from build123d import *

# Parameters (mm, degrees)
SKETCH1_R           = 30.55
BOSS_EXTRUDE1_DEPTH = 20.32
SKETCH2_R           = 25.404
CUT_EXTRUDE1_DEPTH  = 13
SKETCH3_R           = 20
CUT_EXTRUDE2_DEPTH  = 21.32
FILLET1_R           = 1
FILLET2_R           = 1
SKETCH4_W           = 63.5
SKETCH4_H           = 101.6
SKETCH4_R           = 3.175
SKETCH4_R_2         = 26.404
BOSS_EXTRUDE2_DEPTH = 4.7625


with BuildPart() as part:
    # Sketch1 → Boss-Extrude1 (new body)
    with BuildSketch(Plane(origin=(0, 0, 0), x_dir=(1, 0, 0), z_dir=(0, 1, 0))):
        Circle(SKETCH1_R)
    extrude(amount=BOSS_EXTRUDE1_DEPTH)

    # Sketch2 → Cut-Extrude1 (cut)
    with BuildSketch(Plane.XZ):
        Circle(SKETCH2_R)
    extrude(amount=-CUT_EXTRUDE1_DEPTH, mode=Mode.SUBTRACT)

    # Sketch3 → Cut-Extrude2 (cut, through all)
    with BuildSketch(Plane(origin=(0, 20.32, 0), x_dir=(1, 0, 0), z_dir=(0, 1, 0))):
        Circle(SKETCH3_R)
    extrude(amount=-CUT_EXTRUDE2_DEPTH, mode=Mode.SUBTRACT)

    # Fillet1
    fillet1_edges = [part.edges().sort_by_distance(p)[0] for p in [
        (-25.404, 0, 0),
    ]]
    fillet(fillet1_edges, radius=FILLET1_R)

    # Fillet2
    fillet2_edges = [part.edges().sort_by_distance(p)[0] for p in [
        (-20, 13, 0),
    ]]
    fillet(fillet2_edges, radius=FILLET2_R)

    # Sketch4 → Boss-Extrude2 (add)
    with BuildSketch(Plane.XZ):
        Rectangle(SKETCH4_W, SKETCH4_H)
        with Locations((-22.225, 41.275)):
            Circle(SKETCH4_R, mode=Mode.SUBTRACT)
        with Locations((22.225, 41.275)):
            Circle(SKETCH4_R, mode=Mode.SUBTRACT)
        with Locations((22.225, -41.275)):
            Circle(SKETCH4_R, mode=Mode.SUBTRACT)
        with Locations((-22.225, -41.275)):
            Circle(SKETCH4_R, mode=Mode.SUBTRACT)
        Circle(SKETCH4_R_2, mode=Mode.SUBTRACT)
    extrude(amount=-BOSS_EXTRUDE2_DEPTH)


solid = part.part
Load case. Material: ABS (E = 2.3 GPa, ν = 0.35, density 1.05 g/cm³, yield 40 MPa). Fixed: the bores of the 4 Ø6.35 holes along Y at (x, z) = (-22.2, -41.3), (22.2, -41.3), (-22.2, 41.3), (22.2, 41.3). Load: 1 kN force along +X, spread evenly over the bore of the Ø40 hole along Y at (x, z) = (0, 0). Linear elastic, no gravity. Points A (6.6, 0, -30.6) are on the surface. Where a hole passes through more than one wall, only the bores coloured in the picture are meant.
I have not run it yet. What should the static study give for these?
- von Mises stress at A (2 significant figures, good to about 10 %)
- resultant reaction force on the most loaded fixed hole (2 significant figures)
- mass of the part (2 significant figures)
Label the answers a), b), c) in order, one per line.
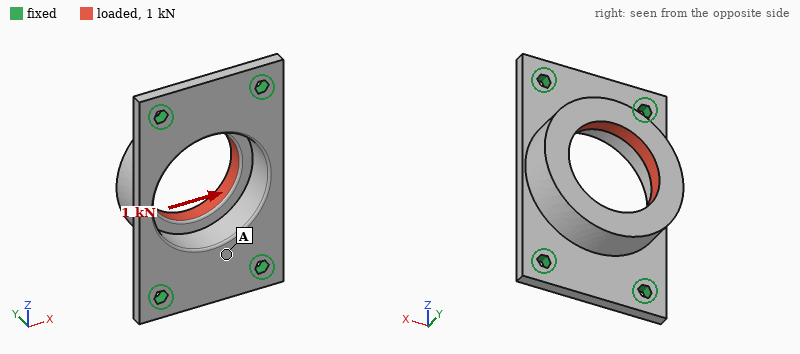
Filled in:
a) 3.5 MPa
b) 340 N
c) 42 g
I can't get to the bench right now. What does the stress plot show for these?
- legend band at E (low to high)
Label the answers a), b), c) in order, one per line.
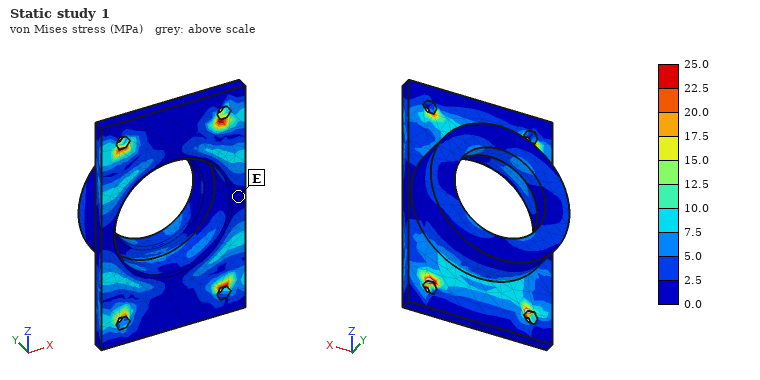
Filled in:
a) 0.0 to 2.5 MPa
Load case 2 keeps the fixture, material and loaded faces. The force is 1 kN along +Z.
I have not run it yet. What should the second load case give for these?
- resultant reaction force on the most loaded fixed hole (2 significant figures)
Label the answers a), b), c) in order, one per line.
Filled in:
a) 270 N
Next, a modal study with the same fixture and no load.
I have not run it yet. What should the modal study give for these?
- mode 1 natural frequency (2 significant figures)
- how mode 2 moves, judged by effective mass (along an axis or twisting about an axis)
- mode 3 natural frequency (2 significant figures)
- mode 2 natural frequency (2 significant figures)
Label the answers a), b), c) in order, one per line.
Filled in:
a) 1400 Hz
b) along Y
c) 2500 Hz
d) 1500 Hz
